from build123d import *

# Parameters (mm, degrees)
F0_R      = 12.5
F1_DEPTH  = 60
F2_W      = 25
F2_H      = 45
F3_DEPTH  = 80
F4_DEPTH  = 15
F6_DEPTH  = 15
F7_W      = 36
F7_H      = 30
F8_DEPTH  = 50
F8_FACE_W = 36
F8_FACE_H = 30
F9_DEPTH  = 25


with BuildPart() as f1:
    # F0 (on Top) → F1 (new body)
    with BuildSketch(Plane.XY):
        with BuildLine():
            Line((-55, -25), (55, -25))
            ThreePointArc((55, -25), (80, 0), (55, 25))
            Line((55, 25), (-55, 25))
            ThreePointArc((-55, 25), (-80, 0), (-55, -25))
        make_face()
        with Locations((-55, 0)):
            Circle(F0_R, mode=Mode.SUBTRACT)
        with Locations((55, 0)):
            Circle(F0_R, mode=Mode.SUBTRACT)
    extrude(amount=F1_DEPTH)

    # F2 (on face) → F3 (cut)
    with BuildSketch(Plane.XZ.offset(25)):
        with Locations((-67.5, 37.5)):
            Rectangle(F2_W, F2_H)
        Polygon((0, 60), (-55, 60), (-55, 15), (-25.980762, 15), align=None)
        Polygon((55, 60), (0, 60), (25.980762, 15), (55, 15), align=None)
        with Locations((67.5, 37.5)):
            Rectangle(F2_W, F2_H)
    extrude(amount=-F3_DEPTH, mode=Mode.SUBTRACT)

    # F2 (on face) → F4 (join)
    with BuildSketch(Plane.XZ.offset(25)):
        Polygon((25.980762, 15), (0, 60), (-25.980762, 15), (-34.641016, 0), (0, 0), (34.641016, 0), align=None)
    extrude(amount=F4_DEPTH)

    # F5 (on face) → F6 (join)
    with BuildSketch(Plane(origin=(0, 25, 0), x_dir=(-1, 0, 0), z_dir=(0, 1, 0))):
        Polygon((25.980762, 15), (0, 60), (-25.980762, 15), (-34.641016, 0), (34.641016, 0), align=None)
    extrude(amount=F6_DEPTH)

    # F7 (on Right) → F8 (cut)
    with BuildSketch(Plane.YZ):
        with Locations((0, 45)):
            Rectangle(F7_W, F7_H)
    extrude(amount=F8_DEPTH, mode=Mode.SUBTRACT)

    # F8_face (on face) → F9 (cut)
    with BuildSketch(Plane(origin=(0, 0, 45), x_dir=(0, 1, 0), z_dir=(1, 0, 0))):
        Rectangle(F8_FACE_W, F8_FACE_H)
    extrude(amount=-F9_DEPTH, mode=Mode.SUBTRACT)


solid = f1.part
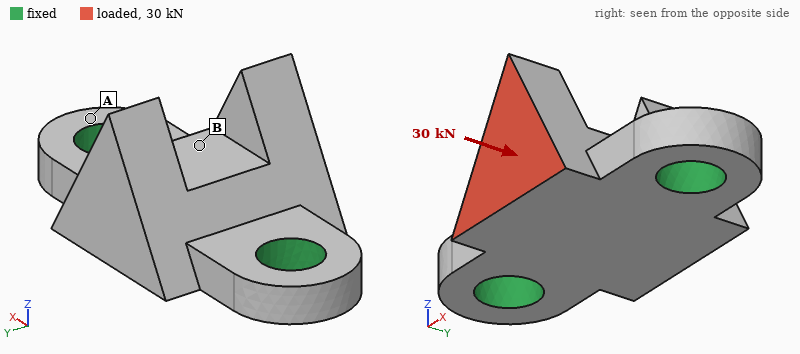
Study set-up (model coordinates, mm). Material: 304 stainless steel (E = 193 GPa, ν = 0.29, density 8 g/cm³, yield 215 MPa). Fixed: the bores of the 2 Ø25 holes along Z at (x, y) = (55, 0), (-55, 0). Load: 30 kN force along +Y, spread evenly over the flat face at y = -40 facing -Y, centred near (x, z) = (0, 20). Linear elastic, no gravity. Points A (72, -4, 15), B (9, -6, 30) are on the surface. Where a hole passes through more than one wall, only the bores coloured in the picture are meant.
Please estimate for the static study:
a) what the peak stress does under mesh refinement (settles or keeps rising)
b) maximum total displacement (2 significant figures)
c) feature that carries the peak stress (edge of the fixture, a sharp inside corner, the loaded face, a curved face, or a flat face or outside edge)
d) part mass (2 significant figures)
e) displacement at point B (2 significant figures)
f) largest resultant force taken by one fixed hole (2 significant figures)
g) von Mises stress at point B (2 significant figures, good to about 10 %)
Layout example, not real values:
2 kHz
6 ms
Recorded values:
keeps rising
92 µm
edge of the fixture
1.6 kg
32 µm
15 kN
35 MPa
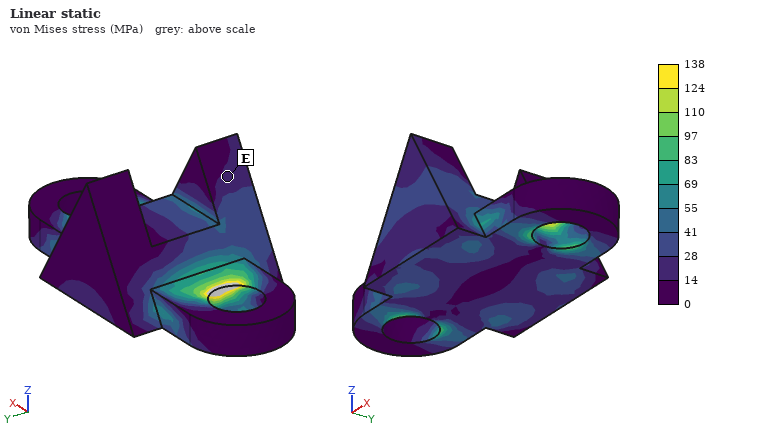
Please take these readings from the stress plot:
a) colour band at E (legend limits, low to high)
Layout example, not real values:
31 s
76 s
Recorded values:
14 to 28 MPa
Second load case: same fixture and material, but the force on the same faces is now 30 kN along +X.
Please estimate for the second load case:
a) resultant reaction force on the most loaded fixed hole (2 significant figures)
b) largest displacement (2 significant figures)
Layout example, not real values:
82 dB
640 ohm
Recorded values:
20 kN
37 µm
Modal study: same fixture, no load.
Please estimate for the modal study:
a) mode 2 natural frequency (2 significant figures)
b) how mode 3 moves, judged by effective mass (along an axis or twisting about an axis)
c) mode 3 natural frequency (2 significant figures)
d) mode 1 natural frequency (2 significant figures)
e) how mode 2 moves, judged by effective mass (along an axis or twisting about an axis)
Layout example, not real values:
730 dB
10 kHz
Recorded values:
5500 Hz
along X
8900 Hz
3200 Hz
along Z
